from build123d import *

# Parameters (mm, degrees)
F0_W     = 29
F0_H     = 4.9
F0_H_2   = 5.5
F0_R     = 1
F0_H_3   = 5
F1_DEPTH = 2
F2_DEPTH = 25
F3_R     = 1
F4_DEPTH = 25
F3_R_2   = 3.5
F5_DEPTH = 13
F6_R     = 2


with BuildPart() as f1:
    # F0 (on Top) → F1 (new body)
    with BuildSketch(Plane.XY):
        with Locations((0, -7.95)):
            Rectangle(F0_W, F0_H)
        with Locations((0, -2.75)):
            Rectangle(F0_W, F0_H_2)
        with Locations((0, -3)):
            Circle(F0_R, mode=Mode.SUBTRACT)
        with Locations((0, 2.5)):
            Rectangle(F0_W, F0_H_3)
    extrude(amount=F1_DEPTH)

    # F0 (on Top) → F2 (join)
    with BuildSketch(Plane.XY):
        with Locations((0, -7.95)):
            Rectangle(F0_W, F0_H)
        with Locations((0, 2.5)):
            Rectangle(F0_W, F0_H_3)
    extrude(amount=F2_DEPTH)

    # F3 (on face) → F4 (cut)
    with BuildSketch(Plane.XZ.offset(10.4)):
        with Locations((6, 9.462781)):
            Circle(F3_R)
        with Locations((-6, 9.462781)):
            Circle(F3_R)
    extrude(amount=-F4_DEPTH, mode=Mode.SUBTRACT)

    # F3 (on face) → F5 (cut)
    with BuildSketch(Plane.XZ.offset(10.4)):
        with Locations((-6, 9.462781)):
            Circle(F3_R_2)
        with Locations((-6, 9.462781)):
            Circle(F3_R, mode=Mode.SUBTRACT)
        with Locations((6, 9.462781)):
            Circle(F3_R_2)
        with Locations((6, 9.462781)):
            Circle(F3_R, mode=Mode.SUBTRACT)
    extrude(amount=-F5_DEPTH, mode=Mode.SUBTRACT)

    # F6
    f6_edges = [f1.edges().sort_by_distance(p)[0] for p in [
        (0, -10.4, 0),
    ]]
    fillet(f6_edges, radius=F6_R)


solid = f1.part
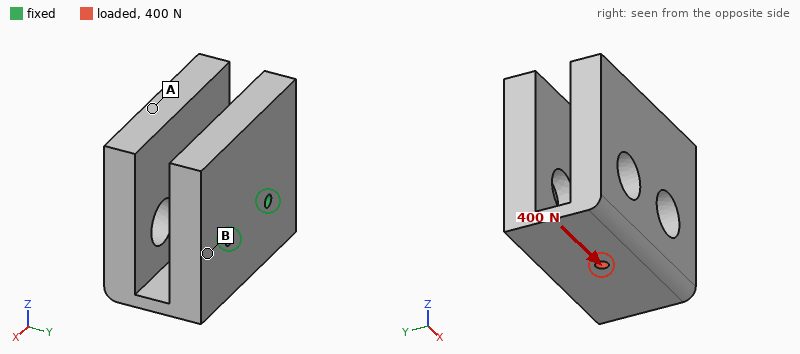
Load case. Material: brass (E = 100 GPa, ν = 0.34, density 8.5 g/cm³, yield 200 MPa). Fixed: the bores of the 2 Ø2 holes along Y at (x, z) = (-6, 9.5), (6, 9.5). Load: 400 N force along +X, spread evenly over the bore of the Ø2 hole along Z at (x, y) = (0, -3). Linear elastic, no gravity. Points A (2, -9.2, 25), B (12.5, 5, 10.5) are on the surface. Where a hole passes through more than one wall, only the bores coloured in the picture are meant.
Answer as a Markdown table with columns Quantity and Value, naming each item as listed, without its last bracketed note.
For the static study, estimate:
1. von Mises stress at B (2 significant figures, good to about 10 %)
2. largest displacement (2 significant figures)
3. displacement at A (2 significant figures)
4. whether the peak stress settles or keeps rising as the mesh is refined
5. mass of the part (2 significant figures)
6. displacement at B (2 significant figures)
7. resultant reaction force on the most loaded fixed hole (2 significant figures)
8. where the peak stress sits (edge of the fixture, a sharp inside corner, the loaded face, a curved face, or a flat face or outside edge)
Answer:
| Quantity | Value |
|---|---|
| von Mises stress at B | 12 MPa |
| largest displacement | 13 µm |
| displacement at A | 11 µm |
| whether the peak stress settles or keeps rising as the mesh is refined | keeps rising |
| mass of the part | 58 g |
| displacement at B | 2.8 µm |
| resultant reaction force on the most loaded fixed hole | 380 N |
| where the peak stress sits | edge of the fixture |
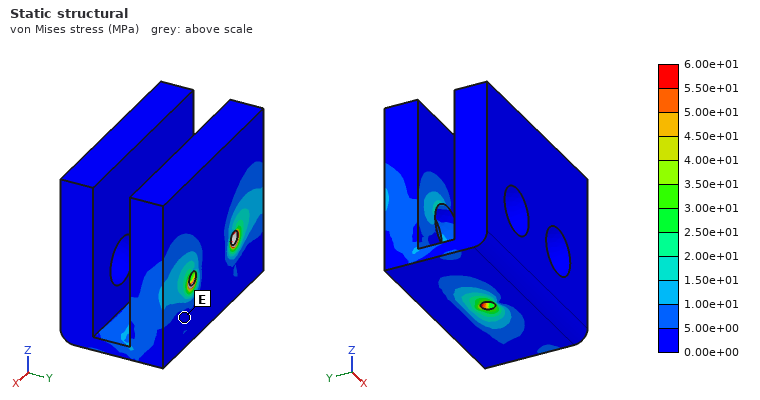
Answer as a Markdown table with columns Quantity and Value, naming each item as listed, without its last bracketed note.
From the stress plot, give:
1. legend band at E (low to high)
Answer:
| Quantity | Value |
|---|---|
| legend band at E | 0.00e+00 to 5.00e+00 MPa |
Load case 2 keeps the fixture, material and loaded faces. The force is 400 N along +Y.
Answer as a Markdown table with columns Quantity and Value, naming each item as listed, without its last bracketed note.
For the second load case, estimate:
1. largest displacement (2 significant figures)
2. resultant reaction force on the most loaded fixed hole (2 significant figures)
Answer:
| Quantity | Value |
|---|---|
| largest displacement | 51 µm |
| resultant reaction force on the most loaded fixed hole | 200 N |
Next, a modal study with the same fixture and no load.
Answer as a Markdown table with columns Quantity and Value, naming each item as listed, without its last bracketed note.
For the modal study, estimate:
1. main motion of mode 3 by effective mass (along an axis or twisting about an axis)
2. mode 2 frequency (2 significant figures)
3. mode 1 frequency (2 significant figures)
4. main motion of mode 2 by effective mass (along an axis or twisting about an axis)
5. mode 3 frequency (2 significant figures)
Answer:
| Quantity | Value |
|---|---|
| main motion of mode 3 by effective mass | along Z |
| mode 2 frequency | 2300 Hz |
| mode 1 frequency | 970 Hz |
| main motion of mode 2 by effective mass | along X |
| mode 3 frequency | 2900 Hz |
